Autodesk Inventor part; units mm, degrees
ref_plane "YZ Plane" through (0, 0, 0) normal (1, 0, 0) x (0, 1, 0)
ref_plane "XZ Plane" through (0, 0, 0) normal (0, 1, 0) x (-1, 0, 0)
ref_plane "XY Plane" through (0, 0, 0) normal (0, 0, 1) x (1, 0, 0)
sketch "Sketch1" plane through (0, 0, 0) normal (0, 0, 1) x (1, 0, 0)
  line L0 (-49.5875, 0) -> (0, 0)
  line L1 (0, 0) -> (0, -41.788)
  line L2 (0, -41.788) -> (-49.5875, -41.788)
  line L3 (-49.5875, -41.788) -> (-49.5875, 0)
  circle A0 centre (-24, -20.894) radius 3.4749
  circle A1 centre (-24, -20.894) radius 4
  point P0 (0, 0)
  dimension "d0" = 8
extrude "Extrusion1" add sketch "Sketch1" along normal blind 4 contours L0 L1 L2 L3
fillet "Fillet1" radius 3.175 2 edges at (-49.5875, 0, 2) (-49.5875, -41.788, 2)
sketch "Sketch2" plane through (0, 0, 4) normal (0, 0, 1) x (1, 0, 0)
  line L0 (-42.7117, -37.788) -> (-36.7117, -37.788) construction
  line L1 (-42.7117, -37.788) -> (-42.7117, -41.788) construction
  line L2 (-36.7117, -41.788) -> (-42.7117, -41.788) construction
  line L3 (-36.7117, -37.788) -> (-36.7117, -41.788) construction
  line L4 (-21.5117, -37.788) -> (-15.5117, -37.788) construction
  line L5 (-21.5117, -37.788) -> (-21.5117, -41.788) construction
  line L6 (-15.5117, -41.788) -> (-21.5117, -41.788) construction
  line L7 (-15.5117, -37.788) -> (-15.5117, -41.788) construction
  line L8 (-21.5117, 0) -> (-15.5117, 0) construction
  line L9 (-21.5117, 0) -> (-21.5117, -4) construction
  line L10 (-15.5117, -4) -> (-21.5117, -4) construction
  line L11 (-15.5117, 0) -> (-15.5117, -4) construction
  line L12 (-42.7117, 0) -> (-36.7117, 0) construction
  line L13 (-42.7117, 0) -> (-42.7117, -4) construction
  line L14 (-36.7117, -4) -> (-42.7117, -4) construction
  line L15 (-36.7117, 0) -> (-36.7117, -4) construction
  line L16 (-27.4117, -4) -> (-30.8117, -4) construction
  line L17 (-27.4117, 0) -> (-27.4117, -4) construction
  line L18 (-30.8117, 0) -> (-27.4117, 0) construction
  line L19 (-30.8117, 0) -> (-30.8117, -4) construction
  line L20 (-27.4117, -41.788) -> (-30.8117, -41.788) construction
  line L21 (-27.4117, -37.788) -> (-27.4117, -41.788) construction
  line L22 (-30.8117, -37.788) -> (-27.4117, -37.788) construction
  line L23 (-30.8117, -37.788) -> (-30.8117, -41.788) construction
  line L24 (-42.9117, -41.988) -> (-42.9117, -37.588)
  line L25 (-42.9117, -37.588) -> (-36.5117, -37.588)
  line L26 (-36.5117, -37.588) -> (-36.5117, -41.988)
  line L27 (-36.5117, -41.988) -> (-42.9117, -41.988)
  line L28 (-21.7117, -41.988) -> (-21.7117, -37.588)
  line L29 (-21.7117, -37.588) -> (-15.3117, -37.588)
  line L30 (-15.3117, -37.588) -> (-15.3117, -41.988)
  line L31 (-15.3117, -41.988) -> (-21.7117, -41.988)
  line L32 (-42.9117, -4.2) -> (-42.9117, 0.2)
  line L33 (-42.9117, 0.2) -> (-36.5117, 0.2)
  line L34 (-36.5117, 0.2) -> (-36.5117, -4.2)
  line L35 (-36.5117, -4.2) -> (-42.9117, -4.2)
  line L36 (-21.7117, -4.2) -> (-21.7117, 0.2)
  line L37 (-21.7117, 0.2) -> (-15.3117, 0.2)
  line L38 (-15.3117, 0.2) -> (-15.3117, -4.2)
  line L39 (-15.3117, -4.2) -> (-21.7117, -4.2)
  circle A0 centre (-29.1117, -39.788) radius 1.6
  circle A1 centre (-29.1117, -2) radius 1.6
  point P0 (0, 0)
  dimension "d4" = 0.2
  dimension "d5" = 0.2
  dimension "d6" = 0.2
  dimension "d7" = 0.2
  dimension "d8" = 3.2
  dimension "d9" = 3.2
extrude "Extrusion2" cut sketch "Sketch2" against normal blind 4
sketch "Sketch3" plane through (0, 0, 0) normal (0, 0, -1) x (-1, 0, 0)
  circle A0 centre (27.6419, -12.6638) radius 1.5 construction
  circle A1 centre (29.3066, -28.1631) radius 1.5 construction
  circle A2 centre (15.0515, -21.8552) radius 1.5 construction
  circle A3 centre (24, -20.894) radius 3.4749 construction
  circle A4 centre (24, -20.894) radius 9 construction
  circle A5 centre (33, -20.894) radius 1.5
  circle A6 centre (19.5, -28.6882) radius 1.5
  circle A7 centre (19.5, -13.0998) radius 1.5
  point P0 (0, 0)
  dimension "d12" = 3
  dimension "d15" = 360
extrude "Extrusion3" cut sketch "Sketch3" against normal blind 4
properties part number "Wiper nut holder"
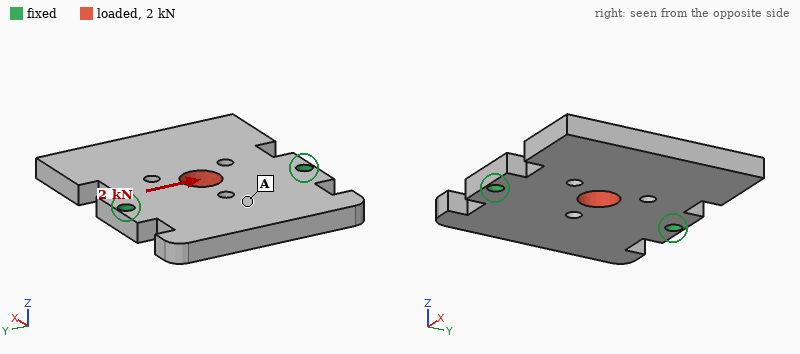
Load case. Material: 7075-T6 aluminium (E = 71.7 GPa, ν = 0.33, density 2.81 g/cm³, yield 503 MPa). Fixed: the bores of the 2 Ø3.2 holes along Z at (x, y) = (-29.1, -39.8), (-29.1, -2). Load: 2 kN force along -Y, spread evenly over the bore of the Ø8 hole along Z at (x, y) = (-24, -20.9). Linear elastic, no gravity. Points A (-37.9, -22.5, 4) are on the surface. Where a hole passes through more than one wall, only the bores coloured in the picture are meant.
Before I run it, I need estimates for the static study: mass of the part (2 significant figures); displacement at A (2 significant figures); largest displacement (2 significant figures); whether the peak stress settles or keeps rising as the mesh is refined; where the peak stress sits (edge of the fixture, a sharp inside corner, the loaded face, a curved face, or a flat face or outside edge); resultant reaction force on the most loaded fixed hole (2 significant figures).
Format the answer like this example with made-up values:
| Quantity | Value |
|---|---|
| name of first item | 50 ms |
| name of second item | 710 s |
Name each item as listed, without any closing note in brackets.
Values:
| Quantity | Value |
|---|---|
| mass of the part | 21 g |
| displacement at A | 2.3 µm |
| largest displacement | 7.9 µm |
| whether the peak stress settles or keeps rising as the mesh is refined | keeps rising |
| where the peak stress sits | edge of the fixture |
| resultant reaction force on the most loaded fixed hole | 1.0 kN |
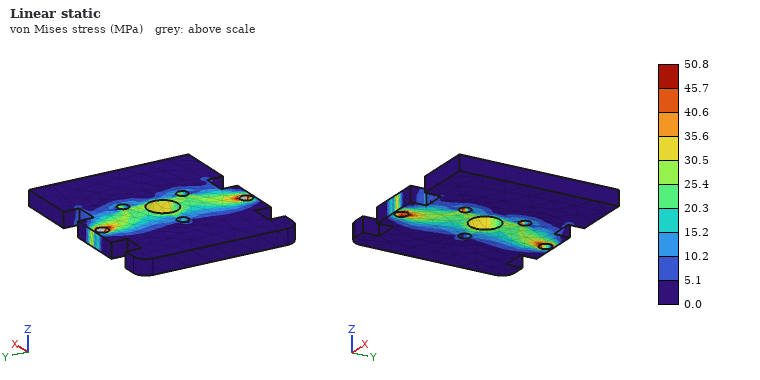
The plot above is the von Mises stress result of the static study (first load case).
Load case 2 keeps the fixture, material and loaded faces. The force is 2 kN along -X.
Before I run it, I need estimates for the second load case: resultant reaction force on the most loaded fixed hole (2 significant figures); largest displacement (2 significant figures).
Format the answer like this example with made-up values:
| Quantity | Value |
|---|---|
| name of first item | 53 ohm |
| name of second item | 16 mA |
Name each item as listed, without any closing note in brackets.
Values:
| Quantity | Value |
|---|---|
| resultant reaction force on the most loaded fixed hole | 1.0 kN |
| largest displacement | 9.5 µm |
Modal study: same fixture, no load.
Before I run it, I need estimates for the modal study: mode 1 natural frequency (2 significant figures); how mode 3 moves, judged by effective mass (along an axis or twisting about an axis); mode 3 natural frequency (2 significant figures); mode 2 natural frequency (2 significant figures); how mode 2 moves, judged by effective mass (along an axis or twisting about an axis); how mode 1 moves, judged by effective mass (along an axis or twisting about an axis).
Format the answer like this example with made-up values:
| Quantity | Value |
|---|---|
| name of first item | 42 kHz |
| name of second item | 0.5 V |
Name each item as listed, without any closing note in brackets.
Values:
| Quantity | Value |
|---|---|
| mode 1 natural frequency | 2700 Hz |
| how mode 3 moves, judged by effective mass | twisting about X |
| mode 3 natural frequency | 6100 Hz |
| mode 2 natural frequency | 5600 Hz |
| how mode 2 moves, judged by effective mass | along Z |
| how mode 1 moves, judged by effective mass | along Z |
